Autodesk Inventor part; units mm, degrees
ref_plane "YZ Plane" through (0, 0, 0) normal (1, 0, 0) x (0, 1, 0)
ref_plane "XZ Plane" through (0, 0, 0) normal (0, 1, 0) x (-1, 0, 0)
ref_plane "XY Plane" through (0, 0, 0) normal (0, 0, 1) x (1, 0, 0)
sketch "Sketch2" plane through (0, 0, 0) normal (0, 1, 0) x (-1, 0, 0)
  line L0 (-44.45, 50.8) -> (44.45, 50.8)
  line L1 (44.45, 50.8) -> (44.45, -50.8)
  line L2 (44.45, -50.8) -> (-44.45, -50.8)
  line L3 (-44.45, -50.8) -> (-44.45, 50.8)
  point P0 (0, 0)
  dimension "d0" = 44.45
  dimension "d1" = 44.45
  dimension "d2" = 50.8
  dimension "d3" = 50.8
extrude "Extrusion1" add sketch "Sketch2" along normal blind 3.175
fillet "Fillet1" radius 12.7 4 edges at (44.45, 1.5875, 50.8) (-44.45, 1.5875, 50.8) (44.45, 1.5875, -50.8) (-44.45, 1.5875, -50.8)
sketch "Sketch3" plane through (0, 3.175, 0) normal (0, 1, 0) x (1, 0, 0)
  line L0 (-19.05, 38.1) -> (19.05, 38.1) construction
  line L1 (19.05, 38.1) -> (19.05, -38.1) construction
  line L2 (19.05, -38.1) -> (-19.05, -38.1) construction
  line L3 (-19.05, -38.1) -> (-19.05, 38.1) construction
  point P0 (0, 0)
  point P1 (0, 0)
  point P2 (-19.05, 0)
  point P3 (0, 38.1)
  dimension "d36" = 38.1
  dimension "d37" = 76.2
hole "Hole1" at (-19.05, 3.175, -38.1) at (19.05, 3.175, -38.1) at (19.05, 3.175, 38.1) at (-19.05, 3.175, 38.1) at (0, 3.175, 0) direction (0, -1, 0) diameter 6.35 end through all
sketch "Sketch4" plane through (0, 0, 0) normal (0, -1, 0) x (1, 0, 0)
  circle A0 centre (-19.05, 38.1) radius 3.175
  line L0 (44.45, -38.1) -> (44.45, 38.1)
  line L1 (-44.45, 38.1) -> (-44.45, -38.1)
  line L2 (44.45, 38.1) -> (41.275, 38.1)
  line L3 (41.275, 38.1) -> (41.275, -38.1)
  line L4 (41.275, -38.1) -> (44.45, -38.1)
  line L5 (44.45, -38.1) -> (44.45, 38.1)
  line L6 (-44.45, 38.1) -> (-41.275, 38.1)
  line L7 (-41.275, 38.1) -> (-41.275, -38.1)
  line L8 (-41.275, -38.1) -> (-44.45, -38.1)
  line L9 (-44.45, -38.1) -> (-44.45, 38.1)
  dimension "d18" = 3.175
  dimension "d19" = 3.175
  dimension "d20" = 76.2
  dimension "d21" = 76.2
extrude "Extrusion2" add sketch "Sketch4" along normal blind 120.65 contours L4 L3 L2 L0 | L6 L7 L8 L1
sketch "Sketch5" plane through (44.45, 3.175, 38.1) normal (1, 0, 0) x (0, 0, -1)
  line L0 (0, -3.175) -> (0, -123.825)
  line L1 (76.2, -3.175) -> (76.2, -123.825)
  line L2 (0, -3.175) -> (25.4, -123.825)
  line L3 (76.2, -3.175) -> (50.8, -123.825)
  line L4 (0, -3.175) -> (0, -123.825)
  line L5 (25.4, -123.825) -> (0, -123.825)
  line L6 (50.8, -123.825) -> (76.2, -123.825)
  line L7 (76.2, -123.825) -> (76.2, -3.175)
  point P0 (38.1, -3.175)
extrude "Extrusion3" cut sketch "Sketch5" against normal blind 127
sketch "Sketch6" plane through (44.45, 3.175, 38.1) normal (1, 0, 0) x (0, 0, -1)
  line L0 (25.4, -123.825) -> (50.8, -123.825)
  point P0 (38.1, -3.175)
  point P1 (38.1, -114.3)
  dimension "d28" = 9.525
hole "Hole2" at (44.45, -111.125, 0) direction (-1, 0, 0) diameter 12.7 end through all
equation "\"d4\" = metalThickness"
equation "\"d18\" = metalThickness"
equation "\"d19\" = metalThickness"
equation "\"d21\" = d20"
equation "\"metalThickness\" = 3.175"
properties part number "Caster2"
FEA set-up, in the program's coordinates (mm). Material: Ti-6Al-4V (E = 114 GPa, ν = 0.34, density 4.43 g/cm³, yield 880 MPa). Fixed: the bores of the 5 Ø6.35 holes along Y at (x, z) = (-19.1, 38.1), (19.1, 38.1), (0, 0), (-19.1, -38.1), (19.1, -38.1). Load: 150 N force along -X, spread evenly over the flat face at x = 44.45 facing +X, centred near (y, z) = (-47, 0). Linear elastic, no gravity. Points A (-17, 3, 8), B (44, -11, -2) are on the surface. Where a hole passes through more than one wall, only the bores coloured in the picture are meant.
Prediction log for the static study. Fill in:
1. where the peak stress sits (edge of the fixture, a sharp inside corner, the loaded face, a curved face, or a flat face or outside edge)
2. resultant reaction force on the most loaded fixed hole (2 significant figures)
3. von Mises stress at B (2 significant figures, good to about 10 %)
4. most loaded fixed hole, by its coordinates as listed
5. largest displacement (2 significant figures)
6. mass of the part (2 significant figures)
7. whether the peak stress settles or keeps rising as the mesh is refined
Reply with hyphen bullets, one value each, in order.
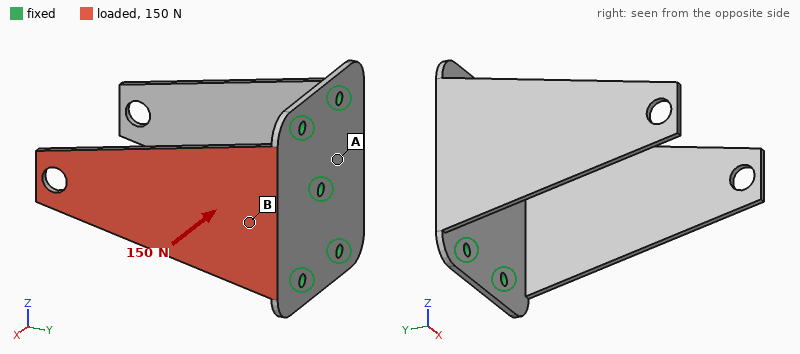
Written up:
- edge of the fixture
- 150 N
- 40 MPa
- (0, 0)
- 1.8 mm
- 290 g
- keeps rising
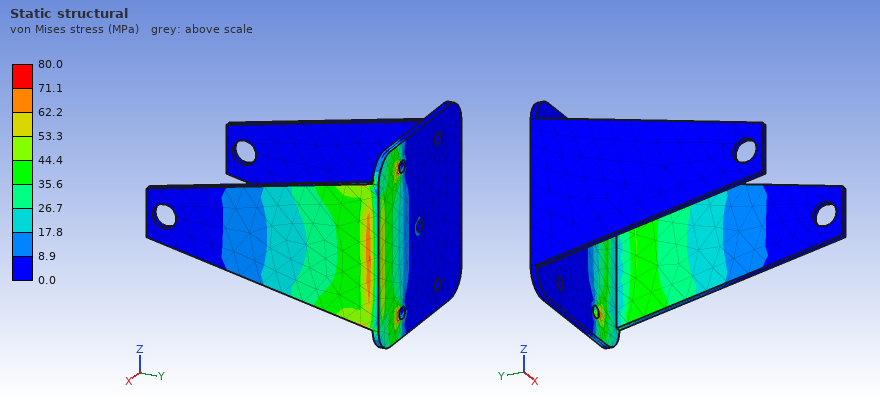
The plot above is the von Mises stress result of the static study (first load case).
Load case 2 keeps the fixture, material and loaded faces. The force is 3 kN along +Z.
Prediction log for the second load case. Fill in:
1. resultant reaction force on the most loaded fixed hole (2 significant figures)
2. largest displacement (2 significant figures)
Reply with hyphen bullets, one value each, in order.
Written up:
- 2.6 kN
- 1.8 mm
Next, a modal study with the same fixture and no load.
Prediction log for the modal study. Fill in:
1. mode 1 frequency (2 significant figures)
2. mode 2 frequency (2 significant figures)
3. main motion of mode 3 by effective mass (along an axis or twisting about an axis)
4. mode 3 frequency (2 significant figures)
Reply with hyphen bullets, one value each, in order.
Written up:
- 210 Hz
- 210 Hz
- along Z
- 830 Hz
